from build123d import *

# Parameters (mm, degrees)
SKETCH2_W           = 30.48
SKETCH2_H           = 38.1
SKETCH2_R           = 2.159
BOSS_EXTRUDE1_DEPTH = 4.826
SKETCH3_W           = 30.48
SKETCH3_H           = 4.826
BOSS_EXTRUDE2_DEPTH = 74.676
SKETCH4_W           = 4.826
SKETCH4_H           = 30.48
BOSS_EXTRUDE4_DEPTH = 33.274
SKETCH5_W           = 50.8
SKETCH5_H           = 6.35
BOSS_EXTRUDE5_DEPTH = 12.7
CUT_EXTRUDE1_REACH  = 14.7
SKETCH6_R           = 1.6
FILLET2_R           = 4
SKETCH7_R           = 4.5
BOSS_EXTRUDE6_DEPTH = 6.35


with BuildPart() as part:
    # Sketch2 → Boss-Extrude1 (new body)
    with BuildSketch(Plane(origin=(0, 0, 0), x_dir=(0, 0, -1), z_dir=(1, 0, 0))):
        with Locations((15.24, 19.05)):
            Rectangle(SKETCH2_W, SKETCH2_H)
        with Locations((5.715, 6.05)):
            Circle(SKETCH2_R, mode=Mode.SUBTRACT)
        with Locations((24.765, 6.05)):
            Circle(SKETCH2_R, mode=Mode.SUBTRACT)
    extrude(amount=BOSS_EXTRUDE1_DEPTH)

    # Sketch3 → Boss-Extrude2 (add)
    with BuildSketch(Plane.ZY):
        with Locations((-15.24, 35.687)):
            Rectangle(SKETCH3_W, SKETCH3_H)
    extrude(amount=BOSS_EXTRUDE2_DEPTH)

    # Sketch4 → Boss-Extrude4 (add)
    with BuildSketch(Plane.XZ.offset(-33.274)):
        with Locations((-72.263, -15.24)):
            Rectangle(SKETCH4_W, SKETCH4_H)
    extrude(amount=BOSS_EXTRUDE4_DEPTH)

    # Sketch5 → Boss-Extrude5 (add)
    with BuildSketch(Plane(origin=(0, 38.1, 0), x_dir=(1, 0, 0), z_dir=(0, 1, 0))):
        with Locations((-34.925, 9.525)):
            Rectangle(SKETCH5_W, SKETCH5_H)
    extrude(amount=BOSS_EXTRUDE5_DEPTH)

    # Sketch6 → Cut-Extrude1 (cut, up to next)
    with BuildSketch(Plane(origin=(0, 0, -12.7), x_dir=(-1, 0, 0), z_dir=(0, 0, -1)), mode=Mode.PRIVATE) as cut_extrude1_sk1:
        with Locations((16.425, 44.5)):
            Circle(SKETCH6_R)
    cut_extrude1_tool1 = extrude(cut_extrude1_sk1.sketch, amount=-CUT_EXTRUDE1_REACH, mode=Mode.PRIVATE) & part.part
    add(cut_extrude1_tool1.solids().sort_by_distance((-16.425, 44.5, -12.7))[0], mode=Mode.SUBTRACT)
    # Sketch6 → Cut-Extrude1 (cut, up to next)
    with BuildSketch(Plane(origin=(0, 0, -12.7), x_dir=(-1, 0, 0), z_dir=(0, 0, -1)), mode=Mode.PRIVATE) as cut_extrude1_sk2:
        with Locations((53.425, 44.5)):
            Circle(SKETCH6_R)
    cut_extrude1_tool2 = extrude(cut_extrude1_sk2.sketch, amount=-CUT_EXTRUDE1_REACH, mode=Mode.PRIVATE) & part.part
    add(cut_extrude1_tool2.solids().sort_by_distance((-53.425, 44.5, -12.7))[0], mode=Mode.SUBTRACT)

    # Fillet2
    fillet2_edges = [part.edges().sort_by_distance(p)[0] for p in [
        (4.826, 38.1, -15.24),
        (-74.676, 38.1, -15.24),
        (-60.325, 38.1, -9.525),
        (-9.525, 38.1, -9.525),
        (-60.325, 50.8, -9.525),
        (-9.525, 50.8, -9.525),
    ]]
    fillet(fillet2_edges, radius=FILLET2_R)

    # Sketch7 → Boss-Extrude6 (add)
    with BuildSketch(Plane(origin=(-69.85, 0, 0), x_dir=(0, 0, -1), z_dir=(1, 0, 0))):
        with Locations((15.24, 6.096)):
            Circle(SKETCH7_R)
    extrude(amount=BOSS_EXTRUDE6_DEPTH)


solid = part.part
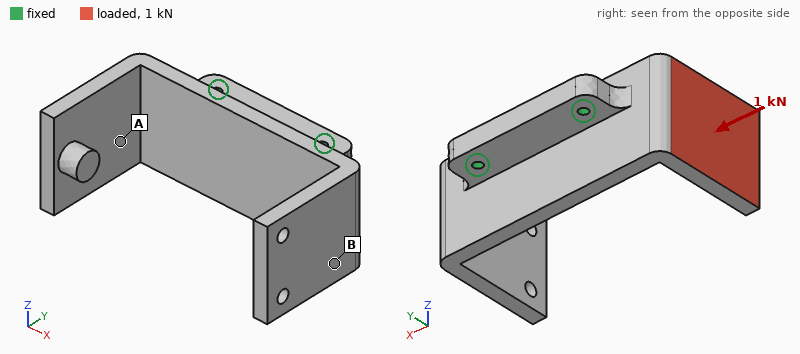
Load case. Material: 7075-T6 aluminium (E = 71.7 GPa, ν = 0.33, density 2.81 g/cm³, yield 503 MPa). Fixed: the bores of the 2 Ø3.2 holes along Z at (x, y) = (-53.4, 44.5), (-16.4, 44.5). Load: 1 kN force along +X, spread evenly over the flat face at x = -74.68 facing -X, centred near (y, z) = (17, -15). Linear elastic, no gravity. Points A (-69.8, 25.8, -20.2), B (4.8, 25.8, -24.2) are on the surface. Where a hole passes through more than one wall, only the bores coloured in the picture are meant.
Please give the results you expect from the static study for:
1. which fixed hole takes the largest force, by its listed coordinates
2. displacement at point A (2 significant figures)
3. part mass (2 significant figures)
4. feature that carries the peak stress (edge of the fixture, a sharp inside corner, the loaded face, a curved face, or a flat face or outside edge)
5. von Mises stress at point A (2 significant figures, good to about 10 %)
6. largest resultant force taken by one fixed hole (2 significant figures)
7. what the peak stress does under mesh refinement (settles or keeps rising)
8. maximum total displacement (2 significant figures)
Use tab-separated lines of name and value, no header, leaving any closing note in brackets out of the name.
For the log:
which fixed hole takes the largest force, by its listed coordinates	(-16.4, 44.5)
displacement at point A	0.20 mm
part mass	72 g
feature that carries the peak stress	a sharp inside corner
von Mises stress at point A	75 MPa
largest resultant force taken by one fixed hole	1.3 kN
what the peak stress does under mesh refinement	keeps rising
maximum total displacement	0.78 mm
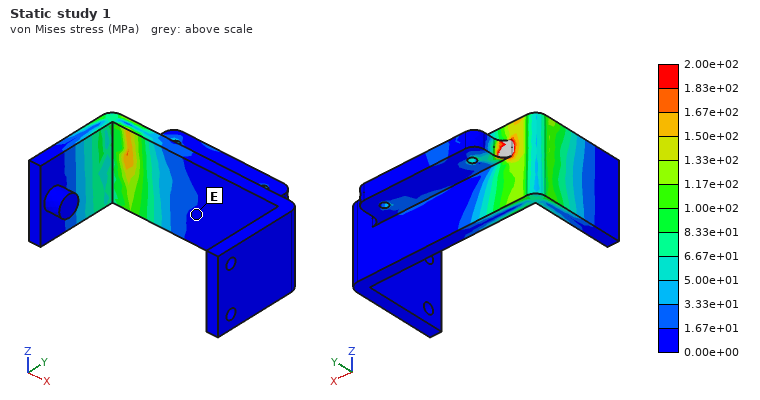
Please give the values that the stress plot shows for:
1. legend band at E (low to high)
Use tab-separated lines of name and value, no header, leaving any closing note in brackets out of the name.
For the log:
legend band at E	0.00e+00 to 1.67e+01 MPa
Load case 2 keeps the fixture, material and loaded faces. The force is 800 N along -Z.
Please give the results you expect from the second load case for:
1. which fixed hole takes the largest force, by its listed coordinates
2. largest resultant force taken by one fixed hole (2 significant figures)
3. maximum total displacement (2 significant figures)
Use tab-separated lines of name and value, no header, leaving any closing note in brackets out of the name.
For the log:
which fixed hole takes the largest force, by its listed coordinates	(-53.4, 44.5)
largest resultant force taken by one fixed hole	1.2 kN
maximum total displacement	0.56 mm
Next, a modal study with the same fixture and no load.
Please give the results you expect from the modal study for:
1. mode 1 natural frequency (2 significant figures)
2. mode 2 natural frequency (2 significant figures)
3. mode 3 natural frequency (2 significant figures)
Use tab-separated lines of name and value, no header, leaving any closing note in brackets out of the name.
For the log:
mode 1 natural frequency	1600 Hz
mode 2 natural frequency	1700 Hz
mode 3 natural frequency	1800 Hz
